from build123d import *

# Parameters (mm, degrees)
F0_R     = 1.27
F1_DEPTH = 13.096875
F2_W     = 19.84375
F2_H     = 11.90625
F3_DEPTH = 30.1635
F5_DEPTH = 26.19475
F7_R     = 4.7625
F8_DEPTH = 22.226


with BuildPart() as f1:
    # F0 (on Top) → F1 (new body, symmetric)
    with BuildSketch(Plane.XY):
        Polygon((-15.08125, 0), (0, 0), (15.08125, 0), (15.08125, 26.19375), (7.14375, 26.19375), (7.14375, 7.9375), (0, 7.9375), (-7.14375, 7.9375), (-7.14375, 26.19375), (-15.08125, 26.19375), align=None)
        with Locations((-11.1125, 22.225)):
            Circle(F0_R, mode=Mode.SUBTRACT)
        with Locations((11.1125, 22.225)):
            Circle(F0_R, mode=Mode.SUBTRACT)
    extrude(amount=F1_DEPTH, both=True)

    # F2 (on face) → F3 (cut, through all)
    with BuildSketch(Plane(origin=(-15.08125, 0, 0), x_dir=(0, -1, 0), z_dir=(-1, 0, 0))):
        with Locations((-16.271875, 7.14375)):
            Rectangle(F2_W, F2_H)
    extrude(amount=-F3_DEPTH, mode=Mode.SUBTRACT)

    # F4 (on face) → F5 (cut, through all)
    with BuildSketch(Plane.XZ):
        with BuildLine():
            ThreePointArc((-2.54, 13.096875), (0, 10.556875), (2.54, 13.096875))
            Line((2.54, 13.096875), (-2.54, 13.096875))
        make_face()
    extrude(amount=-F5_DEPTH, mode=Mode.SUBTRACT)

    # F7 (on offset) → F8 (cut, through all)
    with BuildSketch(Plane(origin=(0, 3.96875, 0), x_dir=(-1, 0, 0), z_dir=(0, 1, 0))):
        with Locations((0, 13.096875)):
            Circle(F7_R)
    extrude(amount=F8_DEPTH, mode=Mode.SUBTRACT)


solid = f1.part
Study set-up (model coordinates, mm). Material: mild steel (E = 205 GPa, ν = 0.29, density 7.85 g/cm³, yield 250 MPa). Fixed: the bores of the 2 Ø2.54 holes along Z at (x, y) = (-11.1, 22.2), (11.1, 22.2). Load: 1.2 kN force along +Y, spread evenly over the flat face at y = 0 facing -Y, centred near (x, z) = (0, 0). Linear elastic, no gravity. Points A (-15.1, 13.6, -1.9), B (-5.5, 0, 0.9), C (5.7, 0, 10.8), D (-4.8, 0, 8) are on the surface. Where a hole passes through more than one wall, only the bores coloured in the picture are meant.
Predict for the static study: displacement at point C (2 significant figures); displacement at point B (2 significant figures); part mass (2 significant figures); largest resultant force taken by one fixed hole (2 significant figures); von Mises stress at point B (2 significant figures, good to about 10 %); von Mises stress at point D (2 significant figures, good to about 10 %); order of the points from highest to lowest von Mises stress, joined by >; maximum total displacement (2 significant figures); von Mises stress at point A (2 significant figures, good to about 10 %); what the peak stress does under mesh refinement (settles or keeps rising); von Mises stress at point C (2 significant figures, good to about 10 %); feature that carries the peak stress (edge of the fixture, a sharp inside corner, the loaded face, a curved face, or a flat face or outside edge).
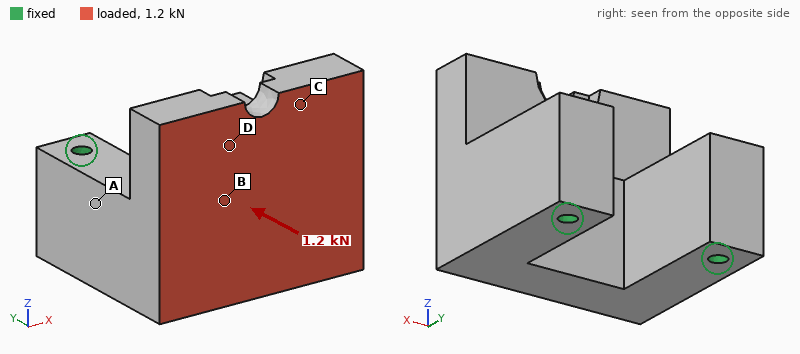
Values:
6.2 µm
3.4 µm
75 g
610 N
13 MPa
5.7 MPa
B > A > D > C
7.1 µm
9.2 MPa
keeps rising
2.8 MPa
edge of the fixture
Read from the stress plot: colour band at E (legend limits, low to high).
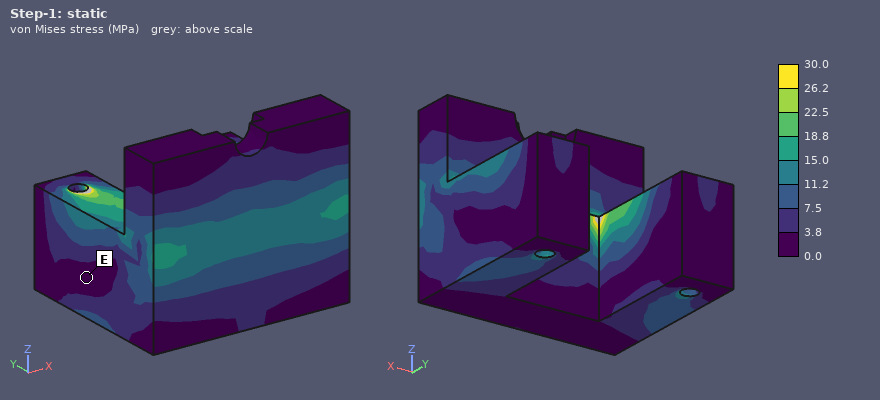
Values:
0.0 to 3.8 MPa
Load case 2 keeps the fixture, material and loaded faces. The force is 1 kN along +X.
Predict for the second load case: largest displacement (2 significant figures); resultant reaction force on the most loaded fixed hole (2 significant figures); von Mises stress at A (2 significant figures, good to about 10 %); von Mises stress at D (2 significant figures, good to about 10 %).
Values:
6.9 µm
830 N
9.3 MPa
7.0 MPa
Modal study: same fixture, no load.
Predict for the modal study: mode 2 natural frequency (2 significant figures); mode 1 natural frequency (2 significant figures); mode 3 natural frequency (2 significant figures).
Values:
10000 Hz
9800 Hz
16 kHz
